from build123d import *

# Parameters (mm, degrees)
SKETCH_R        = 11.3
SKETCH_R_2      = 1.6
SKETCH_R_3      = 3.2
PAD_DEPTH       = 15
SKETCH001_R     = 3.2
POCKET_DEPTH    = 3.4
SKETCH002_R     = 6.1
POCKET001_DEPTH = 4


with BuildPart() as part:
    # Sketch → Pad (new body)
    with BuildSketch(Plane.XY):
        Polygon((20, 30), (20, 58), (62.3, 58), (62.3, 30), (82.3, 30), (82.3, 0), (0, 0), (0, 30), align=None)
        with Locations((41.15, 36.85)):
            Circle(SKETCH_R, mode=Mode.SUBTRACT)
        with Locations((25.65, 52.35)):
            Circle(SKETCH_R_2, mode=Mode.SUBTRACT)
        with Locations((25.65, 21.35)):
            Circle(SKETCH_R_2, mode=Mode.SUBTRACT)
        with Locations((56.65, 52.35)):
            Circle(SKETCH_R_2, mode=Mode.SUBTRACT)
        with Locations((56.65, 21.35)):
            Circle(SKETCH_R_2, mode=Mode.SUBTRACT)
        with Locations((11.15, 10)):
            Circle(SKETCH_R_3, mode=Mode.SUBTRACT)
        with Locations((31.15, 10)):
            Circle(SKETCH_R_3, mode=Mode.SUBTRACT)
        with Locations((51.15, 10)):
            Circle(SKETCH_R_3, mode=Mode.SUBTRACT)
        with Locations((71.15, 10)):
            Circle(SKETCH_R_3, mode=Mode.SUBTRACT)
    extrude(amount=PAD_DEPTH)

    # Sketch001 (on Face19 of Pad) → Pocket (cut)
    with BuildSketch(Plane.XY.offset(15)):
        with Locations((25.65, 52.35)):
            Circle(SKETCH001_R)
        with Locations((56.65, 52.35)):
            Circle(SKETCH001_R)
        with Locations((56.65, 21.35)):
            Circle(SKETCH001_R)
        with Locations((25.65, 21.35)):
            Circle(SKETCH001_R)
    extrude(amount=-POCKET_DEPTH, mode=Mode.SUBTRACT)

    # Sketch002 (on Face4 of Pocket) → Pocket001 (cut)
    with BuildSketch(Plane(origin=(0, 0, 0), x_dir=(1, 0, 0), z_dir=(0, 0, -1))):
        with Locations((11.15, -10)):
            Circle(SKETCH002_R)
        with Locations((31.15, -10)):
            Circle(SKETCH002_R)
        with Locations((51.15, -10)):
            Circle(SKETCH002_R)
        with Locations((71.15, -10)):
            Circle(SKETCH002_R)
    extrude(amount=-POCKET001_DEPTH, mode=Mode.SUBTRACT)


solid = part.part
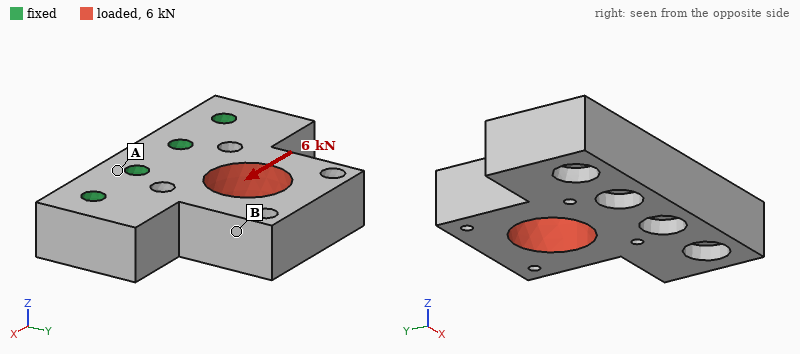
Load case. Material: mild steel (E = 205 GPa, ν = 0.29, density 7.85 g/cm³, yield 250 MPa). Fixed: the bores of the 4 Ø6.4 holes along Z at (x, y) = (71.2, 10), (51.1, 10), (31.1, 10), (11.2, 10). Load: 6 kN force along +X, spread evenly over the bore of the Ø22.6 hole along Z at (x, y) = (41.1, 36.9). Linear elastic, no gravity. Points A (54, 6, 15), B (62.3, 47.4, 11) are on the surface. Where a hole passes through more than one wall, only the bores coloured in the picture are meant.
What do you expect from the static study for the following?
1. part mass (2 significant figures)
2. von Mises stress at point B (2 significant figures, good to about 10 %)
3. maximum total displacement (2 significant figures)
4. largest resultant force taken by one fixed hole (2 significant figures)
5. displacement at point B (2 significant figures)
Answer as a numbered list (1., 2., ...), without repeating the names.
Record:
1. 350 g
2. 17 MPa
3. 9.7 µm
4. 2.8 kN
5. 8.5 µm
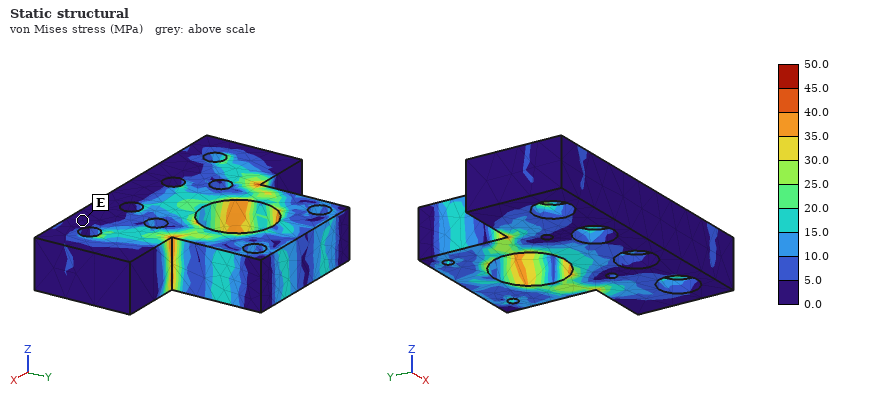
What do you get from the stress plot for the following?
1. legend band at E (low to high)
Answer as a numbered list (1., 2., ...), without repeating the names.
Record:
1. 0.0 to 5.0 MPa
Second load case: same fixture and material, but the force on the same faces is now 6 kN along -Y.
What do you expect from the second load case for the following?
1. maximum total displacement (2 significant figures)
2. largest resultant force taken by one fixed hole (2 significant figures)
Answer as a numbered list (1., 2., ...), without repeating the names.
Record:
1. 3.5 µm
2. 1.9 kN
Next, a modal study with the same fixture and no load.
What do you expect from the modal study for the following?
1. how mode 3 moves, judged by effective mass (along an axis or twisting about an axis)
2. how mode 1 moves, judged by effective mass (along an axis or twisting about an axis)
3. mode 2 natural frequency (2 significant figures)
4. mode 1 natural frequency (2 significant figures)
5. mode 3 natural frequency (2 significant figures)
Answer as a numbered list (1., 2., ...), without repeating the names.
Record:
1. along X
2. along Z
3. 10 kHz
4. 4900 Hz
5. 11 kHz
